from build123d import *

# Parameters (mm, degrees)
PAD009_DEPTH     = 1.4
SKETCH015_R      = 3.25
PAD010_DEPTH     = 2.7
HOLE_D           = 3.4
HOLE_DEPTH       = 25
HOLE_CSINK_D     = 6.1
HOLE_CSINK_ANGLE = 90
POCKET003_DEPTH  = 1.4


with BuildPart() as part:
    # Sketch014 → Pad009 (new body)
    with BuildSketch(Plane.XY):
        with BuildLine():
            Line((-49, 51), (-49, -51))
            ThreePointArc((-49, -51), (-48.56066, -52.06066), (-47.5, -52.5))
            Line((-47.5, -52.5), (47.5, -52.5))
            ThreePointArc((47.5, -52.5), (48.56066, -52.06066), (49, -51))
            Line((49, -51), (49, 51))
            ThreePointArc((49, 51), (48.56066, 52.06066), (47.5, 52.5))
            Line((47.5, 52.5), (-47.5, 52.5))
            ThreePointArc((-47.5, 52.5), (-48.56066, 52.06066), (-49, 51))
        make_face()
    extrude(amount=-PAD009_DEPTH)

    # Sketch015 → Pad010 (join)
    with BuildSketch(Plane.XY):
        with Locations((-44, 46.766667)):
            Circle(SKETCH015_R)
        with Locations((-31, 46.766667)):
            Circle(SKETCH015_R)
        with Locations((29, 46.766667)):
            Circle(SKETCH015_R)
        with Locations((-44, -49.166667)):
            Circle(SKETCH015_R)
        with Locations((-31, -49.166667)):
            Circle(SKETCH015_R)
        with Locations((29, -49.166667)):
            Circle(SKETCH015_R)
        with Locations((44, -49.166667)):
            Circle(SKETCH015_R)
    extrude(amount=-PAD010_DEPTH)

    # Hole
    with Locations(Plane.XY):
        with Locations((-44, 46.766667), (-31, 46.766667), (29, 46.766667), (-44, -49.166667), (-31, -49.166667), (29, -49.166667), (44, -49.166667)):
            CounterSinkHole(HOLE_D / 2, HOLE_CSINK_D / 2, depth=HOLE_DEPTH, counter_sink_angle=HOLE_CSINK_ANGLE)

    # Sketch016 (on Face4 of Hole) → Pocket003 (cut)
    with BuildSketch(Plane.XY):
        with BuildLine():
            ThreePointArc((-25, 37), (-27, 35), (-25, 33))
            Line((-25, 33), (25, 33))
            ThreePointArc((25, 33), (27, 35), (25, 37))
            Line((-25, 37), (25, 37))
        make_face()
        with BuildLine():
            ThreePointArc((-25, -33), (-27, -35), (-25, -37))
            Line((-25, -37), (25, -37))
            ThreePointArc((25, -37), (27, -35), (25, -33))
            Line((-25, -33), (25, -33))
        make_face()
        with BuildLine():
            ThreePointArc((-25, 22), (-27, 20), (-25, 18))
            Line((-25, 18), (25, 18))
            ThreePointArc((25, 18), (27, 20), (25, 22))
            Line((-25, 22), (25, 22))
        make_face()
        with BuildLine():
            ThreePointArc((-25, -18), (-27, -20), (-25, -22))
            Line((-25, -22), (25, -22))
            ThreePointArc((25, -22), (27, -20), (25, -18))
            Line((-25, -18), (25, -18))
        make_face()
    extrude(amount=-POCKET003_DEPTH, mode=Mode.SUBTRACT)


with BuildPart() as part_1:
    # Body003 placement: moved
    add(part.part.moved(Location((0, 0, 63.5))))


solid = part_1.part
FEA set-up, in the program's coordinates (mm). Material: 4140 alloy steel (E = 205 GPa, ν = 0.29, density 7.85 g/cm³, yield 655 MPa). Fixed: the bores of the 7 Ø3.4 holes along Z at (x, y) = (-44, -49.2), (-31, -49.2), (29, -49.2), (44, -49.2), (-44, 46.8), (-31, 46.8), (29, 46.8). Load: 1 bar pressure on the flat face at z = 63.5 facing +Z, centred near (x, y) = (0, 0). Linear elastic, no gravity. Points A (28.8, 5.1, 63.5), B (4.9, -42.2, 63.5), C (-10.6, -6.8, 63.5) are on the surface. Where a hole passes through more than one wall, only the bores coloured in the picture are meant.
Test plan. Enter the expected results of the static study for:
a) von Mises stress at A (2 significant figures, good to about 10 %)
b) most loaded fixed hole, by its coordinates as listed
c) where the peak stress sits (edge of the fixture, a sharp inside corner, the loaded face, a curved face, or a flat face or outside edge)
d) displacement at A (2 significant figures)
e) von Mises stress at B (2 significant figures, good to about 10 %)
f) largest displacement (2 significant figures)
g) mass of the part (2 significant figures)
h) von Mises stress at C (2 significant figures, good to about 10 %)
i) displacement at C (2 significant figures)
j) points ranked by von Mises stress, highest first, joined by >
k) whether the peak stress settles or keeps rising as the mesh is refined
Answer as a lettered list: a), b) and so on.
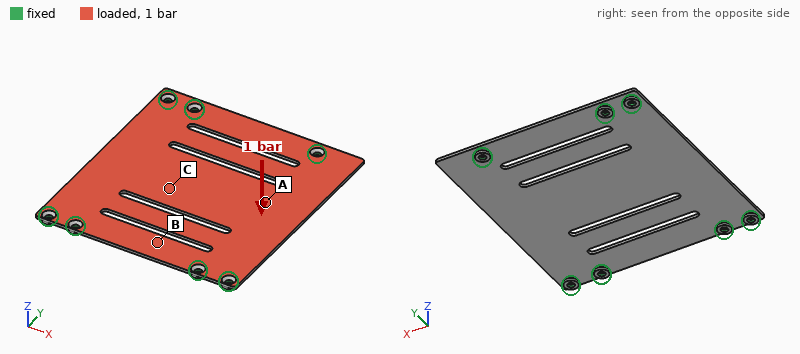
a) 140 MPa
b) (29, 46.8)
c) edge of the fixture
d) 0.72 mm
e) 33 MPa
f) 0.87 mm
g) 100 g
h) 80 MPa
i) 0.84 mm
j) A > C > B
k) keeps rising
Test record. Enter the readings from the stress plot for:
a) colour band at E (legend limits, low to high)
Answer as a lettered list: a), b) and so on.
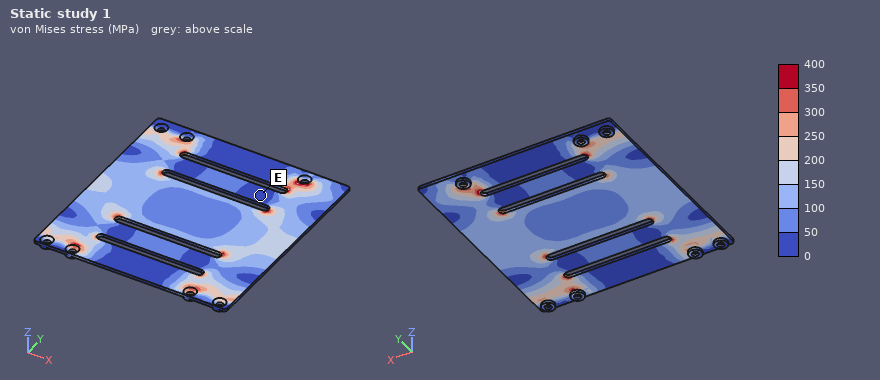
a) 0 to 50 MPa
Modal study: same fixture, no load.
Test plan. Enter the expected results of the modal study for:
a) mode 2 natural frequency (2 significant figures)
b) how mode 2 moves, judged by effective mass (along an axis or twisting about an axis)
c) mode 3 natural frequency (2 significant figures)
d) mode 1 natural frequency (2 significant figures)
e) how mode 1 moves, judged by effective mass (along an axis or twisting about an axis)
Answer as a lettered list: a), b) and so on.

a) 900 Hz
b) twisting about Y
c) 1300 Hz
d) 600 Hz
e) along Z
